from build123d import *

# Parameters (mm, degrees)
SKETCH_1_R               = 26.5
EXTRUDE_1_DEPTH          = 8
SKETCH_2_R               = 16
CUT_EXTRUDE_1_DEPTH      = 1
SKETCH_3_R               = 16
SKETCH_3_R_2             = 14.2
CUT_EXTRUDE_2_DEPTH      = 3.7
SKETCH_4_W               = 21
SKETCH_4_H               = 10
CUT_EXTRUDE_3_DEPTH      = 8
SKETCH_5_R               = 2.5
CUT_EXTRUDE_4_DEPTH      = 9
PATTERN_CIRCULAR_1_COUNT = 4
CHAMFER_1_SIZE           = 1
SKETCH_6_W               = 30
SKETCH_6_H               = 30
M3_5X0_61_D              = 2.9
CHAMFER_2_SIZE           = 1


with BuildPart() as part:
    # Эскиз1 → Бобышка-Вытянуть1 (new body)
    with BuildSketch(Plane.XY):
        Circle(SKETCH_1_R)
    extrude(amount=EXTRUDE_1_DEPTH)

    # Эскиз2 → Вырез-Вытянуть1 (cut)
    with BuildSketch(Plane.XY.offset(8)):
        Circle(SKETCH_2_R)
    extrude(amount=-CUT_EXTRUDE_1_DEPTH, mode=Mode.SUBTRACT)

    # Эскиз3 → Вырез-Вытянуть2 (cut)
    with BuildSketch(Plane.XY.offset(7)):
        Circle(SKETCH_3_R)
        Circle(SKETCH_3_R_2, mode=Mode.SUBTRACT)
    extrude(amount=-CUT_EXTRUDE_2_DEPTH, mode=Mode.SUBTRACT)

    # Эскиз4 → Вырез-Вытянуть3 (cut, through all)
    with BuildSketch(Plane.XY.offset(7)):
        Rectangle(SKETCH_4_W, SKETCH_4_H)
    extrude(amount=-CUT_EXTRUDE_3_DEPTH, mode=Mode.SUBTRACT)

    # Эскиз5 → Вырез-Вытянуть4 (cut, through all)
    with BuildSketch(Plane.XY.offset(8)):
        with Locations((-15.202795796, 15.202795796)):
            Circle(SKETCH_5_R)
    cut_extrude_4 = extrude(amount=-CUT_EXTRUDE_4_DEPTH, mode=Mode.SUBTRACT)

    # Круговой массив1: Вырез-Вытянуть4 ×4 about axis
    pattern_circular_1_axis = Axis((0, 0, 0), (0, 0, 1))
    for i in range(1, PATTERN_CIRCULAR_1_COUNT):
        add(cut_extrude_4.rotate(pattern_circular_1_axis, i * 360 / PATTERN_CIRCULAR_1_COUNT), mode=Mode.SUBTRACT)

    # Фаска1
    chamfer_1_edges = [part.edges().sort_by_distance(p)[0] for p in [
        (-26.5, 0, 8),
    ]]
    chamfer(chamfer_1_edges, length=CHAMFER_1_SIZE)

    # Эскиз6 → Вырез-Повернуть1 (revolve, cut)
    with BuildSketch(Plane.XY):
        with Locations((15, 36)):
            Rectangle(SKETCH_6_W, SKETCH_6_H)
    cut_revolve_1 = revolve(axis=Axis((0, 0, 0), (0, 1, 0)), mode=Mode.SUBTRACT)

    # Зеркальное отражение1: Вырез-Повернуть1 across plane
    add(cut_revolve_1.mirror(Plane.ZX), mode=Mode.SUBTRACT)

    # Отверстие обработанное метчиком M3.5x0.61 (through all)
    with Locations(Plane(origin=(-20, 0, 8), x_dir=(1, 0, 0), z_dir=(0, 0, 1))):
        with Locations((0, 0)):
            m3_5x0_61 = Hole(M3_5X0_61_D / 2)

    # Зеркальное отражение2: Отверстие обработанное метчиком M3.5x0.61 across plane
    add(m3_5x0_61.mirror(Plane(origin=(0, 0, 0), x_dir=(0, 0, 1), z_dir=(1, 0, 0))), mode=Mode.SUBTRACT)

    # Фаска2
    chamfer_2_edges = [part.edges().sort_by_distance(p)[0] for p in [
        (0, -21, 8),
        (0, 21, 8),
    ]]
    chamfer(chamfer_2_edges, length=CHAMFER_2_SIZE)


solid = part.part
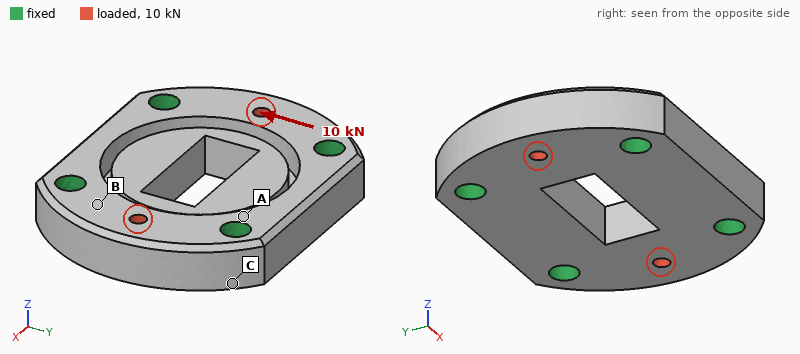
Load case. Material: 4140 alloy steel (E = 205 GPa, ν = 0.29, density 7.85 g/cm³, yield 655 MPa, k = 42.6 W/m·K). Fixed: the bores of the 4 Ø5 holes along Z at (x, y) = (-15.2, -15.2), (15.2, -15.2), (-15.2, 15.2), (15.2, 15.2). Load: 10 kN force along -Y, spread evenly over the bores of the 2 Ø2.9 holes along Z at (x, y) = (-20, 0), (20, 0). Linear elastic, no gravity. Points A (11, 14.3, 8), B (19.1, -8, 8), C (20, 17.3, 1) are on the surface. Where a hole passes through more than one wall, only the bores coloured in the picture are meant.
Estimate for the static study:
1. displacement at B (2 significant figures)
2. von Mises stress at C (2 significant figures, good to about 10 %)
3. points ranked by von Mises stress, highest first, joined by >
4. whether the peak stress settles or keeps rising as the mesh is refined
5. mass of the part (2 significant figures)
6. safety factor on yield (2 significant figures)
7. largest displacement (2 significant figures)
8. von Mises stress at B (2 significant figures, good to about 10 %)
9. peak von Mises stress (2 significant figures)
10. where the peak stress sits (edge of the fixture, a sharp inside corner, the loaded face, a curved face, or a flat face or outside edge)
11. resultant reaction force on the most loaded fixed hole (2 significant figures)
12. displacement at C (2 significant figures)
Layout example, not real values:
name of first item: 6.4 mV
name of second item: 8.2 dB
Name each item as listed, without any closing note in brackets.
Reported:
displacement at B: 1.4 µm
von Mises stress at C: 23 MPa
points ranked by von Mises stress, highest first, joined by >: B > C > A
whether the peak stress settles or keeps rising as the mesh is refined: settles
mass of the part: 94 g
safety factor on yield: 5.3
largest displacement: 3.2 µm
von Mises stress at B: 38 MPa
peak von Mises stress: 120 MPa
where the peak stress sits: the loaded face
resultant reaction force on the most loaded fixed hole: 2.6 kN
displacement at C: 0.57 µm
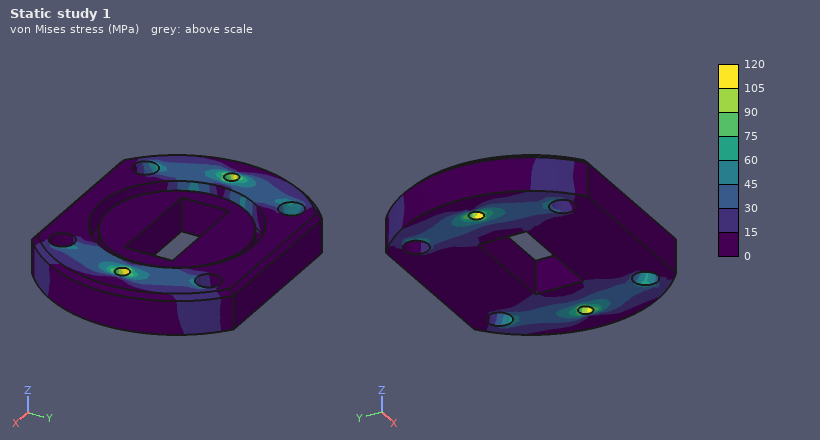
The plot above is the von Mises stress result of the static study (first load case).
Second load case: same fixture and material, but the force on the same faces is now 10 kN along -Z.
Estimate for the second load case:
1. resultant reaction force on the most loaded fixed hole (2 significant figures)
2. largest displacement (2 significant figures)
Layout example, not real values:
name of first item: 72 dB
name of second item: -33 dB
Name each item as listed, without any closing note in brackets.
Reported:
resultant reaction force on the most loaded fixed hole: 2.5 kN
largest displacement: 16 µm
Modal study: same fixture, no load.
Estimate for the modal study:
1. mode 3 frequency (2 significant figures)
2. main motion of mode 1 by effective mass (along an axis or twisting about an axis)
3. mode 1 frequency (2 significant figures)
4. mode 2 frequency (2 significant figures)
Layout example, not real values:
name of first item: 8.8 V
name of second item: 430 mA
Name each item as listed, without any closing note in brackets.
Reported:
mode 3 frequency: 30 kHz
main motion of mode 1 by effective mass: along Z
mode 1 frequency: 26 kHz
mode 2 frequency: 30 kHz
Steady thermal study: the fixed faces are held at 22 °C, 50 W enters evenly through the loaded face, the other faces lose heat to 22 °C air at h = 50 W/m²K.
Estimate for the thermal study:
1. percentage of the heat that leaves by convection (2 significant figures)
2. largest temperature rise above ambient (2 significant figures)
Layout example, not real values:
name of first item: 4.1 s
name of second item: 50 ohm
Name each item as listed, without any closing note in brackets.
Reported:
percentage of the heat that leaves by convection: 6.6 %
largest temperature rise above ambient: 48 K
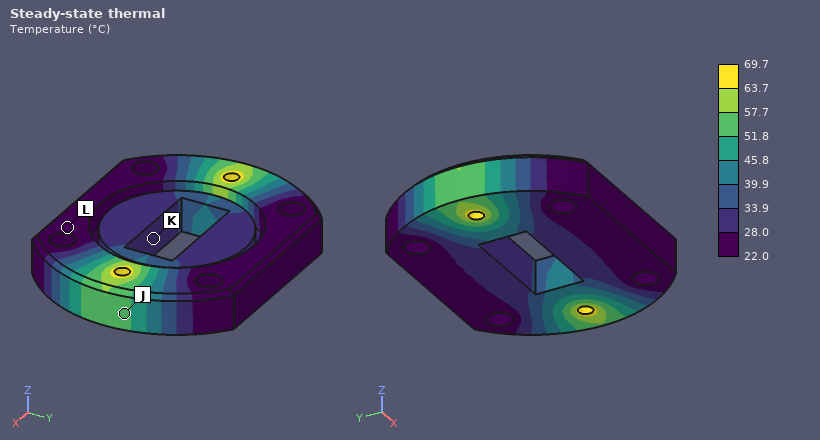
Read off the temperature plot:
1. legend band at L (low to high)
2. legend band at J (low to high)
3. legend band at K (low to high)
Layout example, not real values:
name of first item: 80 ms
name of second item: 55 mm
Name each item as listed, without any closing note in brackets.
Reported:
legend band at L: 22.0 to 28.0 °C
legend band at J: 51.8 to 57.7 °C
legend band at K: 28.0 to 33.9 °C
